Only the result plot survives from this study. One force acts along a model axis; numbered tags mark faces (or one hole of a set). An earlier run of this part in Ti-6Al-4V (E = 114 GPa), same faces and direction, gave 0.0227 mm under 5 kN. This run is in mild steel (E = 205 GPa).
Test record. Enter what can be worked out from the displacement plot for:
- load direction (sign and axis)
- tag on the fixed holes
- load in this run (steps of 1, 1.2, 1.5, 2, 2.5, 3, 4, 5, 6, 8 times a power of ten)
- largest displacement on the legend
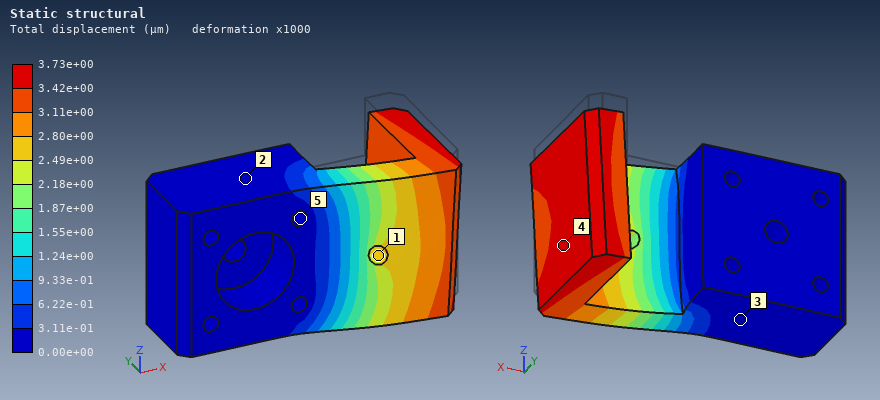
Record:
-Z
5
1.5 kN
3.73e+00 µm
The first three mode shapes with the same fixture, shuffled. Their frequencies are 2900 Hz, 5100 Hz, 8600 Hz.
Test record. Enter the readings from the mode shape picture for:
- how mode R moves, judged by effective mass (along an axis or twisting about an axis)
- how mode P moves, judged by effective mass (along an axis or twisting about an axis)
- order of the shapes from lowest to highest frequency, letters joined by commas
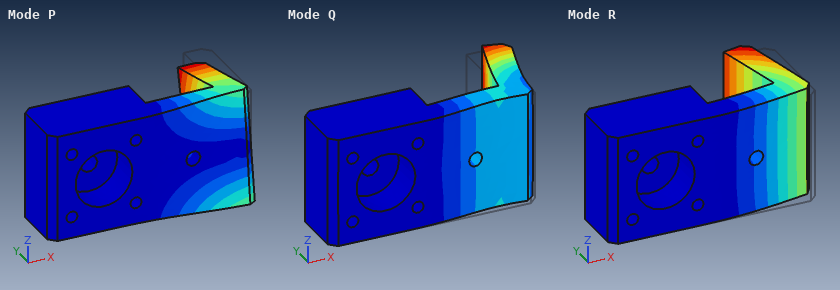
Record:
along Y
along Z
R, P, Q
